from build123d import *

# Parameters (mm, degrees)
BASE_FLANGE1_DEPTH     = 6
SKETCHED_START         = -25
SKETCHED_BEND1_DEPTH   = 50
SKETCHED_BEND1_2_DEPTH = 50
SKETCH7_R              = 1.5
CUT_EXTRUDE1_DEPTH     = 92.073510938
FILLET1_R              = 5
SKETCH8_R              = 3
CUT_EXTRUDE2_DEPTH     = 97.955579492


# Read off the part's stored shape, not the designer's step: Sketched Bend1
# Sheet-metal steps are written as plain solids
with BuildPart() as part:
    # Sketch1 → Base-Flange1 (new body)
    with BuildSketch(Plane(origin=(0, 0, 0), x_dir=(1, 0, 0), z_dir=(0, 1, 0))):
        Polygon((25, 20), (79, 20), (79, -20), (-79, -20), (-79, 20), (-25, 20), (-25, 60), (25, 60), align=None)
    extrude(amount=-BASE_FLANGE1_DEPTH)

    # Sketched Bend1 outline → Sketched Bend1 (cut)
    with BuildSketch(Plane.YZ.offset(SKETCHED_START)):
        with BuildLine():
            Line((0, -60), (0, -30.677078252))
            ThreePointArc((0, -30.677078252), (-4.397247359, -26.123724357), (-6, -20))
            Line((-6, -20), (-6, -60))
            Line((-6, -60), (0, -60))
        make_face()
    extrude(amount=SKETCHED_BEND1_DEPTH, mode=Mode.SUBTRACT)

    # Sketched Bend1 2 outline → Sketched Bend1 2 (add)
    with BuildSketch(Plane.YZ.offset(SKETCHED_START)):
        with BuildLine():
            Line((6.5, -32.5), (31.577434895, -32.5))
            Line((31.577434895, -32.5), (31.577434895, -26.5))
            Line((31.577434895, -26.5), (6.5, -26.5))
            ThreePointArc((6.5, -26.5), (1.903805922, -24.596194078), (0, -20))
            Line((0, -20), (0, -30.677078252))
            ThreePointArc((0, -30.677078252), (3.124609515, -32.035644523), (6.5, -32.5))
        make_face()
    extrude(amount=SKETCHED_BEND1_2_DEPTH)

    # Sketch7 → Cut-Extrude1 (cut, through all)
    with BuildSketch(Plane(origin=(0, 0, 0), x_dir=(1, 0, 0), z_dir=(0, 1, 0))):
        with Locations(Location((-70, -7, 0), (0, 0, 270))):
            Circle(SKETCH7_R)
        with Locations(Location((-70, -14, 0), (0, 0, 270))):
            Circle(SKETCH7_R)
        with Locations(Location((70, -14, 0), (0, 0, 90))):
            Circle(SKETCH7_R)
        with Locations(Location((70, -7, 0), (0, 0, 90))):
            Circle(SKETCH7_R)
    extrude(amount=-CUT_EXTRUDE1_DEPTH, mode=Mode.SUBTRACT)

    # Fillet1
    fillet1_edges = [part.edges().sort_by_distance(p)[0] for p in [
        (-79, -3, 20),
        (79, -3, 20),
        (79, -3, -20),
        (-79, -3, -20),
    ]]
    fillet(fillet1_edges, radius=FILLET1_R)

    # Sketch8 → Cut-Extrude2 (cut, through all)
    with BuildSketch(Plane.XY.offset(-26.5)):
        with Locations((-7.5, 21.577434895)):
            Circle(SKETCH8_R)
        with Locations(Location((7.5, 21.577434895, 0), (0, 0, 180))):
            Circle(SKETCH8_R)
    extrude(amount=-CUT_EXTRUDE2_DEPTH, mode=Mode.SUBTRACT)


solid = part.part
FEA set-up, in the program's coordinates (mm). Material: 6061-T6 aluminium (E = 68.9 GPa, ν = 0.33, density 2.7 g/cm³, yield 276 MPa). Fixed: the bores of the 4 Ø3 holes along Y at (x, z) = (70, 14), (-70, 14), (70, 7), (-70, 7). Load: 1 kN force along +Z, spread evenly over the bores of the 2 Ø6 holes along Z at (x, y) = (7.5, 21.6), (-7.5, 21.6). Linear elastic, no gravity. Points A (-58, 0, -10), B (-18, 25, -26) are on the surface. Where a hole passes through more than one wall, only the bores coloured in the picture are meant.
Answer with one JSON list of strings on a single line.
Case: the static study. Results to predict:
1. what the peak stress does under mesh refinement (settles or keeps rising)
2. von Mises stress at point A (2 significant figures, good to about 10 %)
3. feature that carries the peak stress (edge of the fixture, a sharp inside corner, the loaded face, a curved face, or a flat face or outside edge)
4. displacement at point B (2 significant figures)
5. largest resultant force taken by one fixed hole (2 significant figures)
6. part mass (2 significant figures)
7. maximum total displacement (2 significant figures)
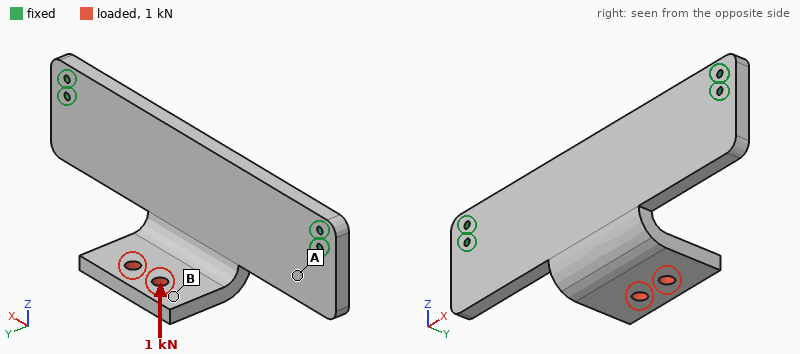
["keeps rising", "36 MPa", "edge of the fixture", "0.62 mm", "1.0 kN", "130 g", "0.82 mm"]
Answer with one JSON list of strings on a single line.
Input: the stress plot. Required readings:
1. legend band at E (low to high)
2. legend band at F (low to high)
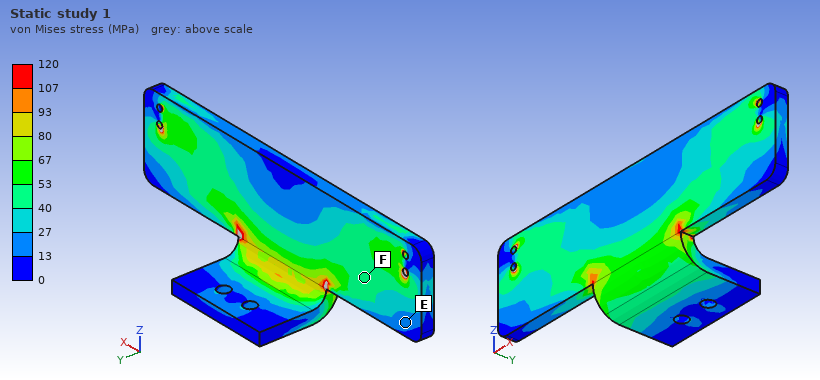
["13 to 27 MPa", "40 to 53 MPa"]
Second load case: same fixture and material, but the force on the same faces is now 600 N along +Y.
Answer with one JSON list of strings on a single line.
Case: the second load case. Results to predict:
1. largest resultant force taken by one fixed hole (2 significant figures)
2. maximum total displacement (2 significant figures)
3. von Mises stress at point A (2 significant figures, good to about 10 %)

["880 N", "0.55 mm", "30 MPa"]
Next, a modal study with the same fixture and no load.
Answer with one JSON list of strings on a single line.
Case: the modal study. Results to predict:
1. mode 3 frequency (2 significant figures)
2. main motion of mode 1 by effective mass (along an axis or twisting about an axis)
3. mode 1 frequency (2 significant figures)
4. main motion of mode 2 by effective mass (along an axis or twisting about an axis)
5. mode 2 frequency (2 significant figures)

["2300 Hz", "along Y", "890 Hz", "along Y", "1700 Hz"]
